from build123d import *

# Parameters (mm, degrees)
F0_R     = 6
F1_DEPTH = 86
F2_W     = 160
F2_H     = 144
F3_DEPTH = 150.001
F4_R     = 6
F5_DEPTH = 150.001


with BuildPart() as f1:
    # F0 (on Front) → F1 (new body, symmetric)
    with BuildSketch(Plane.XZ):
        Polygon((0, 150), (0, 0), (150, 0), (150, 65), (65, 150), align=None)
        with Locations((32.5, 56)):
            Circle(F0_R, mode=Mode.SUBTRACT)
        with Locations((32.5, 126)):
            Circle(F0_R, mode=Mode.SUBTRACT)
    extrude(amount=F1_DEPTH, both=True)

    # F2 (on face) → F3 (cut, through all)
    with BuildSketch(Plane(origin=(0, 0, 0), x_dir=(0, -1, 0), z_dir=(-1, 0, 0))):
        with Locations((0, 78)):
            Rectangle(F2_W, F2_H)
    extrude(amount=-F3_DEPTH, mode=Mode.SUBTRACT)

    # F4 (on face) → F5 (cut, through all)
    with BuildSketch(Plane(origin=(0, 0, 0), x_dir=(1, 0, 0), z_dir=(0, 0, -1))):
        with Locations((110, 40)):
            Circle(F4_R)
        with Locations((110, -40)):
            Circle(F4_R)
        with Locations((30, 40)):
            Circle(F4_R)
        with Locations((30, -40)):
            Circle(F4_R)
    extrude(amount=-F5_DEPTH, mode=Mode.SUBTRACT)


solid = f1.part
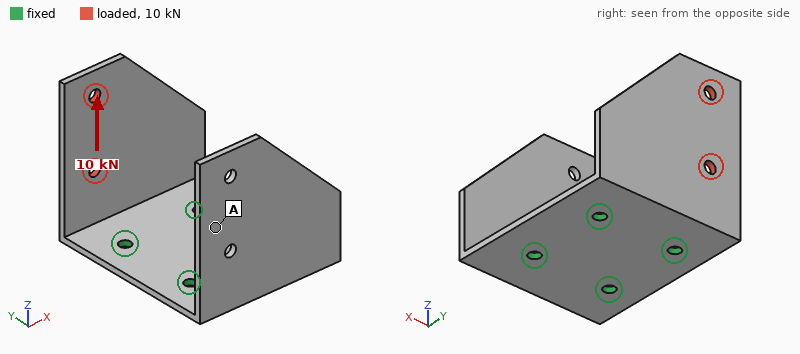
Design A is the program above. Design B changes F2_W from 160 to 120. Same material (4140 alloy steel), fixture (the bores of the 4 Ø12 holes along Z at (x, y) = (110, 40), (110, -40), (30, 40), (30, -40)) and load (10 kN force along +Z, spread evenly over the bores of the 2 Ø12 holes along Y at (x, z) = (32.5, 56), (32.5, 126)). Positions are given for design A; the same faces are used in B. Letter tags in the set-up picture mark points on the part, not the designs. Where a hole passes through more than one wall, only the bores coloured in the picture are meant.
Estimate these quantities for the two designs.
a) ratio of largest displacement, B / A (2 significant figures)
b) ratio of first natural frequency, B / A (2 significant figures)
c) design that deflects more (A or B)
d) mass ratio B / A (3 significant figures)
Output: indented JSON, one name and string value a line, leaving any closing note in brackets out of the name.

{
  "ratio of largest displacement, B / A": "0.44",
  "ratio of first natural frequency, B / A": "0.84",
  "design that deflects more": "A",
  "mass ratio B / A": "2.95"
}
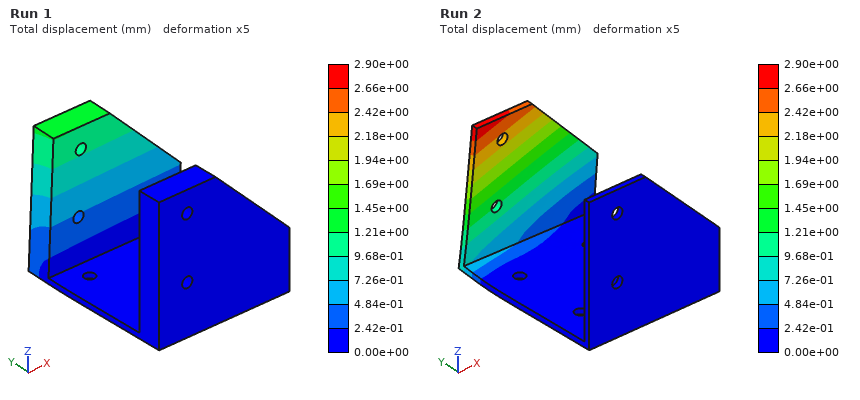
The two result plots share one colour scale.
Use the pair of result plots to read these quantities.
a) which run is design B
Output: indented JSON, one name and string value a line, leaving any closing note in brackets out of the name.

{
  "which run is design B": "Run 1"
}
